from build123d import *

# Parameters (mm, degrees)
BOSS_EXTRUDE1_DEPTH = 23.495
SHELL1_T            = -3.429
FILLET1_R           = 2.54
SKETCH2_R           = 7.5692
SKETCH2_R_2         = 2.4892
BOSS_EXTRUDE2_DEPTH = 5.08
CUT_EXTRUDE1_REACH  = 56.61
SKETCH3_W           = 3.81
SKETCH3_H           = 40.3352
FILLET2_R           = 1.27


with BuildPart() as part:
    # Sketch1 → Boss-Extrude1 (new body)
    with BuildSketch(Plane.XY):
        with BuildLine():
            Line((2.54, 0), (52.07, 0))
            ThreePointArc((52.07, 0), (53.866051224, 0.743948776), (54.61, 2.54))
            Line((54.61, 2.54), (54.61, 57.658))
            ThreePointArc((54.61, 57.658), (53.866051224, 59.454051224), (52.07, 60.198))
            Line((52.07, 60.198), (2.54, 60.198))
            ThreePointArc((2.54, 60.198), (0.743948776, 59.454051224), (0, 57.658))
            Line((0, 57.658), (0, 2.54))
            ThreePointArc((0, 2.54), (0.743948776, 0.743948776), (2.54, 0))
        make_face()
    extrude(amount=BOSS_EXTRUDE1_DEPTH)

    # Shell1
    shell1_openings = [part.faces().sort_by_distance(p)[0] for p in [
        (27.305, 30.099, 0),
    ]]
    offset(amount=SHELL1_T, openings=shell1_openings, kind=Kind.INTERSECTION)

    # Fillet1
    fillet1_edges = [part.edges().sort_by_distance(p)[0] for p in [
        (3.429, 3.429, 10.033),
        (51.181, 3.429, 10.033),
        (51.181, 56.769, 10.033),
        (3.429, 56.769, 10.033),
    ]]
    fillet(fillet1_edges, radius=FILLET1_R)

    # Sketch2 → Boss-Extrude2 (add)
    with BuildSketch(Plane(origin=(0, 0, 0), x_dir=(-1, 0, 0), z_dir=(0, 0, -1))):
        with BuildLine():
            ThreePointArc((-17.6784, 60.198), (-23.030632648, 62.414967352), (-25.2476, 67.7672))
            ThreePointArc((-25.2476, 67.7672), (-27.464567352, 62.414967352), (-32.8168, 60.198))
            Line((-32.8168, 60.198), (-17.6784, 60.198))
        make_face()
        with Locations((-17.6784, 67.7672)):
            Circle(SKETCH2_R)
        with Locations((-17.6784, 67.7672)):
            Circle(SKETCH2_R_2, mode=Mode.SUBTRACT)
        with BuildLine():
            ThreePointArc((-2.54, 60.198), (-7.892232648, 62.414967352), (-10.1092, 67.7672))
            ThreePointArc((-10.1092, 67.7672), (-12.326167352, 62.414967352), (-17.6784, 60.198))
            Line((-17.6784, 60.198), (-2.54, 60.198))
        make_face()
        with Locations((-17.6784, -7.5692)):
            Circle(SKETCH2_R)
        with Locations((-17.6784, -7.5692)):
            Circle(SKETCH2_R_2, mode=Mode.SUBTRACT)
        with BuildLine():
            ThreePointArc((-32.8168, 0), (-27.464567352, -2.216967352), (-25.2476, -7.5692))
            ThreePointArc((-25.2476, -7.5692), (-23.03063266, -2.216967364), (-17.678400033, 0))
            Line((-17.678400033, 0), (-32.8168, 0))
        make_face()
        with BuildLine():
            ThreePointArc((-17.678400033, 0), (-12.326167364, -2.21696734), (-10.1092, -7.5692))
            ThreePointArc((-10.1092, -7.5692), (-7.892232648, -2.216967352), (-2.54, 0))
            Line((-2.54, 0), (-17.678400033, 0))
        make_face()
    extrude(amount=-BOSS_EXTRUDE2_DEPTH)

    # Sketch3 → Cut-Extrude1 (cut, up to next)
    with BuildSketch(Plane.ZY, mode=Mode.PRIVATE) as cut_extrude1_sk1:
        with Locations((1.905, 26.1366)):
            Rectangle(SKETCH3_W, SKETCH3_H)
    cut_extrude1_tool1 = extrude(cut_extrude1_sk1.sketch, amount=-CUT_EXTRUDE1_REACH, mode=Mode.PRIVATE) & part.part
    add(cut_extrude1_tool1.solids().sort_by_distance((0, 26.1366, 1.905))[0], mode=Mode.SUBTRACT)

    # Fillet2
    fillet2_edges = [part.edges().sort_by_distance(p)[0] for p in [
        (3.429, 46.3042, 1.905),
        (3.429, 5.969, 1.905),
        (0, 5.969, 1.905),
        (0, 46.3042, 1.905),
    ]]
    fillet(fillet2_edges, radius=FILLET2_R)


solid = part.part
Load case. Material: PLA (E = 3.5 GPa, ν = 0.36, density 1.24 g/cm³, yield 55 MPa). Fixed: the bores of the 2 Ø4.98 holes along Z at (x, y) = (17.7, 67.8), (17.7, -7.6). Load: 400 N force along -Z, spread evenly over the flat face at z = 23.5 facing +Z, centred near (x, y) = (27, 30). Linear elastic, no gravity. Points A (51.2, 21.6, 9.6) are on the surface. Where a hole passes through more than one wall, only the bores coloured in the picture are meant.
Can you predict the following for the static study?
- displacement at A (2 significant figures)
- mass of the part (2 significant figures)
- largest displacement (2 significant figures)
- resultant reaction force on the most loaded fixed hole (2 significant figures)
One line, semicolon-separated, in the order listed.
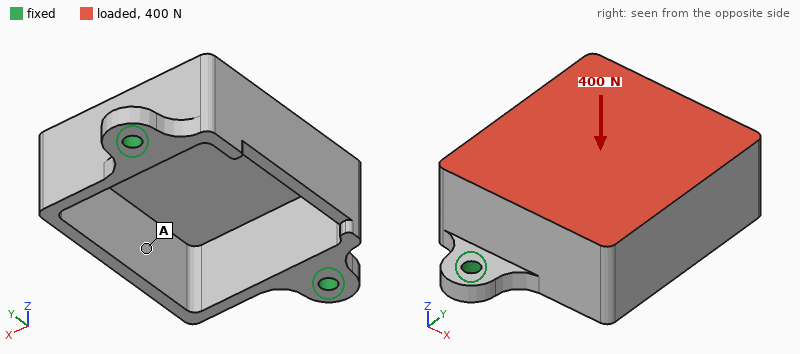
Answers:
0.64 mm; 34 g; 0.74 mm; 210 N
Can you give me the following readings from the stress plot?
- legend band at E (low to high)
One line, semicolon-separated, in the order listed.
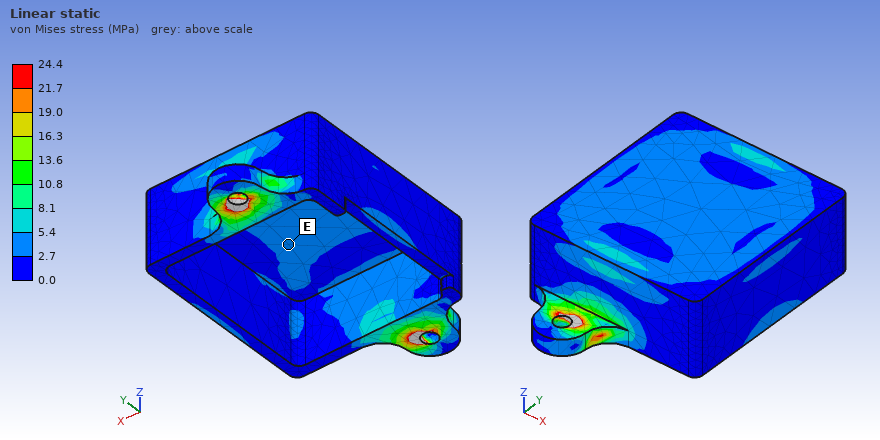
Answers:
2.7 to 5.4 MPa
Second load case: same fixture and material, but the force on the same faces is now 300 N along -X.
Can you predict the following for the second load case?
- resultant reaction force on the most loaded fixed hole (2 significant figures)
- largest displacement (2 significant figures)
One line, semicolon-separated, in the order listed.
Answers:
150 N; 1.1 mm
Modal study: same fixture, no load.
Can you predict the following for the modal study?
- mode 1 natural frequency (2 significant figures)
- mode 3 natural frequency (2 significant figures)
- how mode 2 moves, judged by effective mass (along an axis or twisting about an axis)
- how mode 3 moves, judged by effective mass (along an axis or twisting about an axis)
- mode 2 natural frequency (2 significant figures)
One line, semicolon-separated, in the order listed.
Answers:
530 Hz; 1800 Hz; along Y; along Y; 850 Hz
